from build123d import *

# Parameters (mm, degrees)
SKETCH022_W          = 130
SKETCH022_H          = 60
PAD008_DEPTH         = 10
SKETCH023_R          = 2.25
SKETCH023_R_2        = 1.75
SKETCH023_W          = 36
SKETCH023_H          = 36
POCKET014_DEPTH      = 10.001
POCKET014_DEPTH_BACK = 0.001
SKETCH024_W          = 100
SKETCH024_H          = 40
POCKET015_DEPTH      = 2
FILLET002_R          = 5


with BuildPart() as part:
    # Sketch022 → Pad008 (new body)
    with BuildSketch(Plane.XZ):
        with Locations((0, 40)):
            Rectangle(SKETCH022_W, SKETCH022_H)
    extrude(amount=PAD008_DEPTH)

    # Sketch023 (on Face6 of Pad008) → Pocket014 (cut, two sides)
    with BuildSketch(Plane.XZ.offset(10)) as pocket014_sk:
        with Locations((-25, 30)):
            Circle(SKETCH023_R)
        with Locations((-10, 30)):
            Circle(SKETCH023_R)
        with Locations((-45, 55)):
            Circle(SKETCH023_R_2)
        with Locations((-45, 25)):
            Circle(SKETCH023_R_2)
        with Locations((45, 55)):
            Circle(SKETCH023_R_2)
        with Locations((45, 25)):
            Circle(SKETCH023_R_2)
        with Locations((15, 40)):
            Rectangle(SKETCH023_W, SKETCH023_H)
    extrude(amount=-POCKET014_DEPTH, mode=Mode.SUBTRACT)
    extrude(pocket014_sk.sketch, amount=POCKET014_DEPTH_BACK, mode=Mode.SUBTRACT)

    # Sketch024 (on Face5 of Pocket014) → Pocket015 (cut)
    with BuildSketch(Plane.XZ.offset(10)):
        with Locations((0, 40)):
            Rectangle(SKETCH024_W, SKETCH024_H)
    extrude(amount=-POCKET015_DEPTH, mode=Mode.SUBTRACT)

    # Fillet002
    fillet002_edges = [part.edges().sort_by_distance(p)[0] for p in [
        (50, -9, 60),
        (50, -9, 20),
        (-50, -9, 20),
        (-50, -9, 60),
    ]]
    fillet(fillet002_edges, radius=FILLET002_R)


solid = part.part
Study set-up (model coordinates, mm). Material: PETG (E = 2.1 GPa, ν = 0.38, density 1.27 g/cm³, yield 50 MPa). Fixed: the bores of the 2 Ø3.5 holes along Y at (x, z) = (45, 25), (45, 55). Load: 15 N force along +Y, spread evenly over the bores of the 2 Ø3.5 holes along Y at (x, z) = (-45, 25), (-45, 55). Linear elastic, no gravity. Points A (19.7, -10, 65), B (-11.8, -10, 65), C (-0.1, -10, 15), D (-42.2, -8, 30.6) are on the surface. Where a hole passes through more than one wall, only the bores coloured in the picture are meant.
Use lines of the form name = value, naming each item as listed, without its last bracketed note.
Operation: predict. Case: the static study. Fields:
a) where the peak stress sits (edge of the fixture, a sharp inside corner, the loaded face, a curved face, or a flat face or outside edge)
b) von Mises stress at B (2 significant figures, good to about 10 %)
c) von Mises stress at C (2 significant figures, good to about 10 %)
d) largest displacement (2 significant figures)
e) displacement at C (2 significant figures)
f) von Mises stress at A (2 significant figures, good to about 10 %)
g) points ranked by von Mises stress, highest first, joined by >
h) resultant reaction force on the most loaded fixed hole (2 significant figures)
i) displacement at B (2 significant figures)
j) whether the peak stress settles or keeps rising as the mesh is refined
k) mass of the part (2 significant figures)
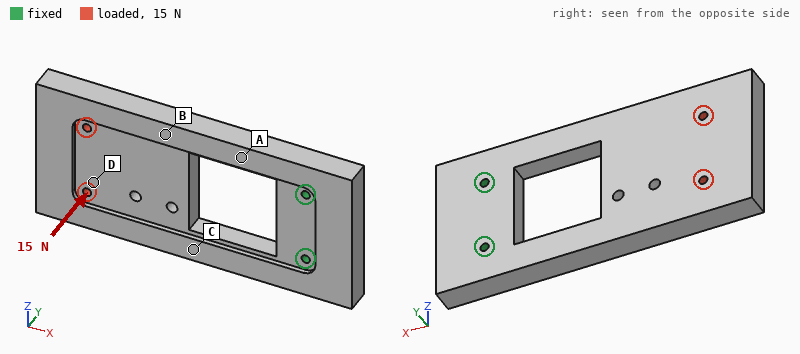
where the peak stress sits = edge of the fixture
von Mises stress at B = 1.0 MPa
von Mises stress at C = 1.8 MPa
largest displacement = 1.3 mm
displacement at C = 0.34 mm
von Mises stress at A = 2.7 MPa
points ranked by von Mises stress, highest first, joined by > = A > C > B > D
resultant reaction force on the most loaded fixed hole = 7.9 N
displacement at B = 0.50 mm
whether the peak stress settles or keeps rising as the mesh is refined = keeps rising
mass of the part = 75 g
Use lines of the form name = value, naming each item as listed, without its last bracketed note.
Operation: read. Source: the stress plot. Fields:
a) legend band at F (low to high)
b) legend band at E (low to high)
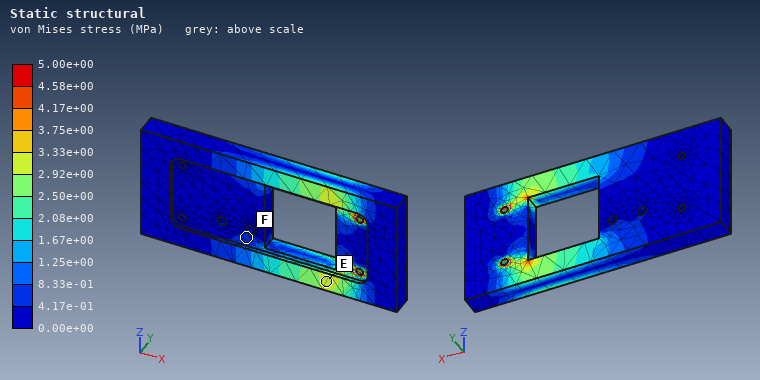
legend band at F = 4.17e-01 to 8.33e-01 MPa
legend band at E = 2.92e+00 to 3.33e+00 MPa
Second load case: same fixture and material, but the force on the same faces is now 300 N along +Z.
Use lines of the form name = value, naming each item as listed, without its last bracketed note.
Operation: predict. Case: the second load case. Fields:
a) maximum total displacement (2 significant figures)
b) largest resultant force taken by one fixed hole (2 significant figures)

maximum total displacement = 1.4 mm
largest resultant force taken by one fixed hole = 840 N
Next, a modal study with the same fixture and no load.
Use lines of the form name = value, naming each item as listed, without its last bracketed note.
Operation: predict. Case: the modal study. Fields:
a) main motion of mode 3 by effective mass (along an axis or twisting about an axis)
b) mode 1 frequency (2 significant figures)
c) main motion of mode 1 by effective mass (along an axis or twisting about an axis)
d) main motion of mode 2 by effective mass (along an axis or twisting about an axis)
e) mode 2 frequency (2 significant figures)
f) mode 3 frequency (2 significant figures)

main motion of mode 3 by effective mass = along Z
mode 1 frequency = 110 Hz
main motion of mode 1 by effective mass = along Y
main motion of mode 2 by effective mass = along Z
mode 2 frequency = 380 Hz
mode 3 frequency = 410 Hz
